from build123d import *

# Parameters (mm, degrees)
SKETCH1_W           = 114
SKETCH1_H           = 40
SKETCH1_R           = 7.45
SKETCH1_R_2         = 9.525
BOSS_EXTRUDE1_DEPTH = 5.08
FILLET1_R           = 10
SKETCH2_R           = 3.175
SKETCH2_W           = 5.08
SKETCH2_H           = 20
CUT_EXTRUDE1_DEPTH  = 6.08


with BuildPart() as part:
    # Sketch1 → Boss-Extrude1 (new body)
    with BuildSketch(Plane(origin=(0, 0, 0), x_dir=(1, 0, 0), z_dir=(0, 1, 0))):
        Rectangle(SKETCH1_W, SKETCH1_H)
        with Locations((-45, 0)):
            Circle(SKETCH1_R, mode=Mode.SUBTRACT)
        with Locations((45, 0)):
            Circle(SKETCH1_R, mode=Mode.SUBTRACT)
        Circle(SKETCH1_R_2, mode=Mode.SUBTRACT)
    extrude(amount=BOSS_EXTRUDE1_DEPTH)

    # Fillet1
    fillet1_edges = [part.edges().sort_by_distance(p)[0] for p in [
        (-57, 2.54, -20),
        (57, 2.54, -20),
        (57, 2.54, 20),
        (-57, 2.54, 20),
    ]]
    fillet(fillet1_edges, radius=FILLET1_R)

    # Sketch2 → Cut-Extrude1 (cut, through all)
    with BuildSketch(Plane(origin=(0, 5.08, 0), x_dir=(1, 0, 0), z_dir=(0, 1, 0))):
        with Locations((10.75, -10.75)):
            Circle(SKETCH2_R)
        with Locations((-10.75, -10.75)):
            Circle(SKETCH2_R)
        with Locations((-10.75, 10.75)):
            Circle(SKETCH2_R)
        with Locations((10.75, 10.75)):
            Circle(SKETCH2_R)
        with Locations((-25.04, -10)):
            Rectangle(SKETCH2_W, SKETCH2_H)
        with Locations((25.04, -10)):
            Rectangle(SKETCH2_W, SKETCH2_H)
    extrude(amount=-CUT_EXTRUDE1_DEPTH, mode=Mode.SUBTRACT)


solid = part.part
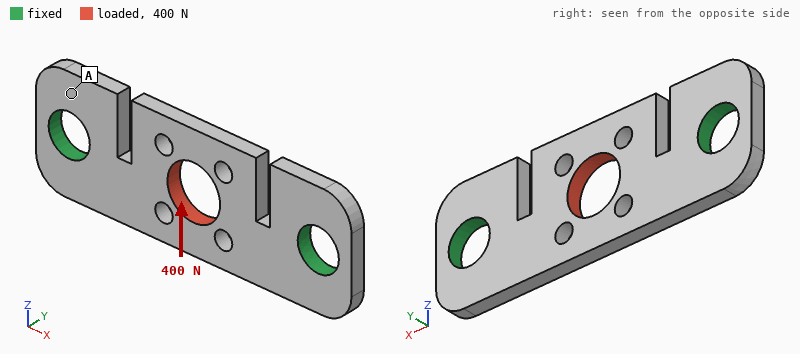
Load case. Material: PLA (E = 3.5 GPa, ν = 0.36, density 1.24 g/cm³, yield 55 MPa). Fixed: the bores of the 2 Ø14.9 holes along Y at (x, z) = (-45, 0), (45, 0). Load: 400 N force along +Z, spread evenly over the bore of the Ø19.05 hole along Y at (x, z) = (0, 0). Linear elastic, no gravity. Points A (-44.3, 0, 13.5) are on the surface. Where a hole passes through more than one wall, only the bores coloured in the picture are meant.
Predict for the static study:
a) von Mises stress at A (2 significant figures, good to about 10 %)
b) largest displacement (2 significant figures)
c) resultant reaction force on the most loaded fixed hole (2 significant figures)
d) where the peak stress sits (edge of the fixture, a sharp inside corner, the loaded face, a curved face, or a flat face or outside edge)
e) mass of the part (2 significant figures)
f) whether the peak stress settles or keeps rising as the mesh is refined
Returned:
0.84 MPa
94 µm
210 N
a sharp inside corner
22 g
keeps rising
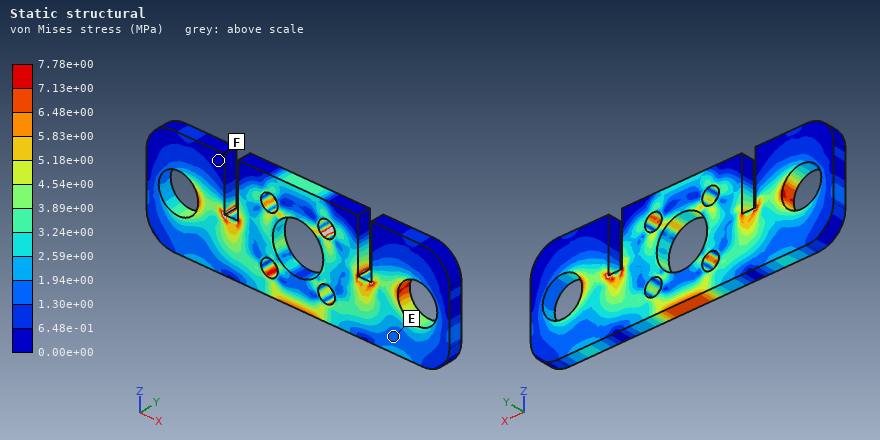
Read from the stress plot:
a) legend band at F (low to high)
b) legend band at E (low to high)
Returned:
0.00e+00 to 6.48e-01 MPa
1.30e+00 to 1.94e+00 MPa
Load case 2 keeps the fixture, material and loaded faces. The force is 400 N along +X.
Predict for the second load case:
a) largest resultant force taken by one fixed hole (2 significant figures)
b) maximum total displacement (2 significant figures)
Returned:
200 N
58 µm
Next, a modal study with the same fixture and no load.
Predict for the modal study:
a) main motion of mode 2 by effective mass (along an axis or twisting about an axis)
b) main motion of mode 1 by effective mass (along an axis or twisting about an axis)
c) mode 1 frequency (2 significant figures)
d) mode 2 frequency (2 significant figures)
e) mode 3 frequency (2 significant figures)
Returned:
along Y
along Y
920 Hz
1500 Hz
2200 Hz
